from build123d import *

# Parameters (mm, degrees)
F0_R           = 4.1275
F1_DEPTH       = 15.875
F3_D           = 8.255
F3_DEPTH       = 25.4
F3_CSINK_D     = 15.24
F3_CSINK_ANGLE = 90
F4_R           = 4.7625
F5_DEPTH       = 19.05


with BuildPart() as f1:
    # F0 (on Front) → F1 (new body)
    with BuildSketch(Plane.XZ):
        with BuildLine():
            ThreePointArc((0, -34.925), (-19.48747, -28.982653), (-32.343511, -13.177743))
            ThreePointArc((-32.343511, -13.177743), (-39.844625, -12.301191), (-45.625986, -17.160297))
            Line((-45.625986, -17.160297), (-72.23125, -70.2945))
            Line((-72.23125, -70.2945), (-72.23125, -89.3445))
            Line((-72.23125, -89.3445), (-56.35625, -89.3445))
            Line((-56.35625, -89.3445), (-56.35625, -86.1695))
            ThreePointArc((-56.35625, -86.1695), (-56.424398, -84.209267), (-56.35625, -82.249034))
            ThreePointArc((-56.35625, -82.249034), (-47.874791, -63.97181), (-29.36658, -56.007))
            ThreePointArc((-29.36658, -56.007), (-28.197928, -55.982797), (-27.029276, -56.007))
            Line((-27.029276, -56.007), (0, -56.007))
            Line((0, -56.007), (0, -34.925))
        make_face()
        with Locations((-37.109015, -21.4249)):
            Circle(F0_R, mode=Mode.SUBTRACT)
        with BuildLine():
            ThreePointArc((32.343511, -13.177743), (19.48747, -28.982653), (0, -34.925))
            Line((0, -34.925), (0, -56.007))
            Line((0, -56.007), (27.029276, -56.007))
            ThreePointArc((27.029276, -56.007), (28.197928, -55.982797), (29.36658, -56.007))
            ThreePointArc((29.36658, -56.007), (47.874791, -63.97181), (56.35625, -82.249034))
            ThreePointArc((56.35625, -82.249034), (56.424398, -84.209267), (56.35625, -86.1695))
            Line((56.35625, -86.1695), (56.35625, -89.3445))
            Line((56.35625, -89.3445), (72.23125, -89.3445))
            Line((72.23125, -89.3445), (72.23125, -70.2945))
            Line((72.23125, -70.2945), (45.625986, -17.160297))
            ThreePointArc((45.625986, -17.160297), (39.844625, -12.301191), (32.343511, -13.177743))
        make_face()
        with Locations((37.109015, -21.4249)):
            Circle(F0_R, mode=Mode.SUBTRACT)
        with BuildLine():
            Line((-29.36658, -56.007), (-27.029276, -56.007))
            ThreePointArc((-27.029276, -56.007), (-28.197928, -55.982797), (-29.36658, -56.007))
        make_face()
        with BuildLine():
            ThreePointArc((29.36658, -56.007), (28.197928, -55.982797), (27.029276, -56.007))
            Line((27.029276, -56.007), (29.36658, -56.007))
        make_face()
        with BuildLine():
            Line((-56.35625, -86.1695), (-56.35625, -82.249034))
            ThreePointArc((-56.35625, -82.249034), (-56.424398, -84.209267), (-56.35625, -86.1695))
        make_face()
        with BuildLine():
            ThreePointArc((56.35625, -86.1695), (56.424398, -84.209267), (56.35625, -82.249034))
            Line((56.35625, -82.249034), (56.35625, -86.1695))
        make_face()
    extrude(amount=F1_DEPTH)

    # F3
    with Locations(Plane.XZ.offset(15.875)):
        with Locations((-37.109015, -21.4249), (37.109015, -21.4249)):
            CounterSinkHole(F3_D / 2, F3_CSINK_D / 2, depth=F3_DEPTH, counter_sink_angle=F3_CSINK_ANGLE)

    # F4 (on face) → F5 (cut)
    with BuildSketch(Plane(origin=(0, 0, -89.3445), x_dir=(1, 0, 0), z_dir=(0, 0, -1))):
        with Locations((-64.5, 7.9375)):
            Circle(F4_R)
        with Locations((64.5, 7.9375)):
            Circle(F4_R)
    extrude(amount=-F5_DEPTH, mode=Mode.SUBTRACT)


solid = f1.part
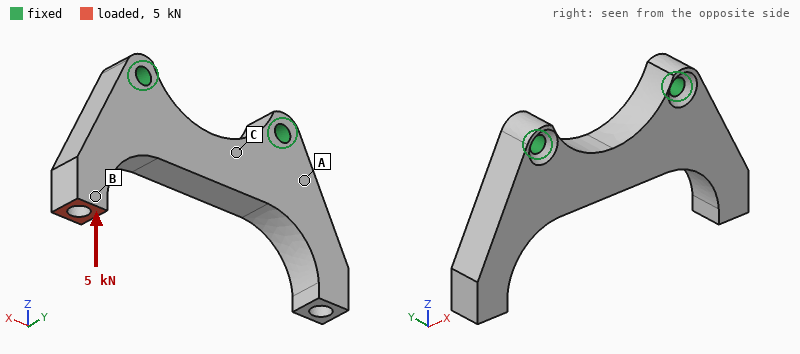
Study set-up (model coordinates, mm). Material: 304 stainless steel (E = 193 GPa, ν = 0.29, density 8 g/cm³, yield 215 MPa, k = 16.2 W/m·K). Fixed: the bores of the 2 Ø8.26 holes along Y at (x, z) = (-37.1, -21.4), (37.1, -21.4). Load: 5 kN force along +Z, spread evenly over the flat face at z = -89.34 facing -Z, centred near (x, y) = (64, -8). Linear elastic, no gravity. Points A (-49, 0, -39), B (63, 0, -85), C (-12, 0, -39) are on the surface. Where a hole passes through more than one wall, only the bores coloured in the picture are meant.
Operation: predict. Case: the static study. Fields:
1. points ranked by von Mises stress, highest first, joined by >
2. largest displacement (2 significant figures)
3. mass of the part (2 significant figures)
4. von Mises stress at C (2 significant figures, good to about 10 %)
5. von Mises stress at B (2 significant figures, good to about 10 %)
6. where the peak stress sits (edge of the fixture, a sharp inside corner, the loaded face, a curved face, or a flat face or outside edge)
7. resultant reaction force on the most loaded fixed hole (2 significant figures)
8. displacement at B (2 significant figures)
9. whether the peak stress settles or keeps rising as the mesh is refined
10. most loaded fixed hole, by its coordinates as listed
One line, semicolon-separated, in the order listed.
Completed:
B > C > A; 53 µm; 590 g; 12 MPa; 27 MPa; edge of the fixture; 6.7 kN; 43 µm; keeps rising; (37.1, -21.4)
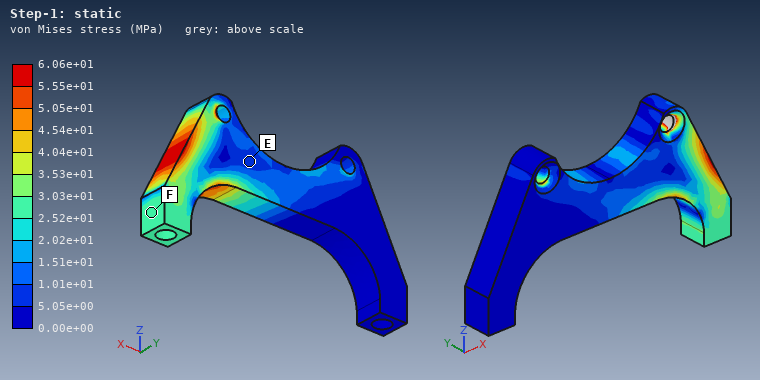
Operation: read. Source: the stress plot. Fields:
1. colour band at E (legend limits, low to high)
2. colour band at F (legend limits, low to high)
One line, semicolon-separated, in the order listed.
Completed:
5.05e+00 to 1.01e+01 MPa; 2.52e+01 to 3.03e+01 MPa
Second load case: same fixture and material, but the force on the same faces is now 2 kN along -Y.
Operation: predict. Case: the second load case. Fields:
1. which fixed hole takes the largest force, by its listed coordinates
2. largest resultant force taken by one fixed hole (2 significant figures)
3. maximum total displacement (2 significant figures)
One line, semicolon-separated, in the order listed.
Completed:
(37.1, -21.4); 2.3 kN; 0.19 mm
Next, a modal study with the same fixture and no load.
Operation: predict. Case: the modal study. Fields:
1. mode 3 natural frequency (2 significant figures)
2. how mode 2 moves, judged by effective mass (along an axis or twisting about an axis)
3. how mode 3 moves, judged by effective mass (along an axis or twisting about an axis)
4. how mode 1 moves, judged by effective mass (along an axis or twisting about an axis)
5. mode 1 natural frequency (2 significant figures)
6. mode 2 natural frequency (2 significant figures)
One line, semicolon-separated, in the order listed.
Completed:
5300 Hz; twisting about Z; along X; along Y; 2800 Hz; 3000 Hz
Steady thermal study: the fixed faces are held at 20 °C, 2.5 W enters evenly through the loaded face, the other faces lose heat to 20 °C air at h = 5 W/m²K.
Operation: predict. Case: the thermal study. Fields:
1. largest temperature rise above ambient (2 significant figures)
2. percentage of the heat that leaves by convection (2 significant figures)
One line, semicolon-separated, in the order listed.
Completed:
34 K; 19 %
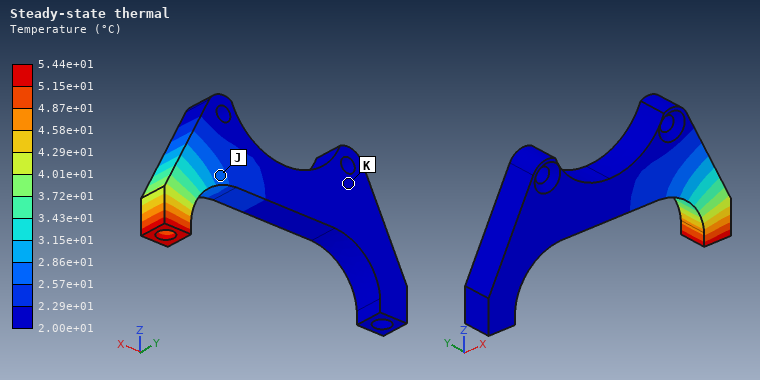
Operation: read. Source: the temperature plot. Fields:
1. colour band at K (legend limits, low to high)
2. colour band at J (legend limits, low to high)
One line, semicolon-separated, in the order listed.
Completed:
2.00e+01 to 2.29e+01 °C; 2.57e+01 to 2.86e+01 °C
